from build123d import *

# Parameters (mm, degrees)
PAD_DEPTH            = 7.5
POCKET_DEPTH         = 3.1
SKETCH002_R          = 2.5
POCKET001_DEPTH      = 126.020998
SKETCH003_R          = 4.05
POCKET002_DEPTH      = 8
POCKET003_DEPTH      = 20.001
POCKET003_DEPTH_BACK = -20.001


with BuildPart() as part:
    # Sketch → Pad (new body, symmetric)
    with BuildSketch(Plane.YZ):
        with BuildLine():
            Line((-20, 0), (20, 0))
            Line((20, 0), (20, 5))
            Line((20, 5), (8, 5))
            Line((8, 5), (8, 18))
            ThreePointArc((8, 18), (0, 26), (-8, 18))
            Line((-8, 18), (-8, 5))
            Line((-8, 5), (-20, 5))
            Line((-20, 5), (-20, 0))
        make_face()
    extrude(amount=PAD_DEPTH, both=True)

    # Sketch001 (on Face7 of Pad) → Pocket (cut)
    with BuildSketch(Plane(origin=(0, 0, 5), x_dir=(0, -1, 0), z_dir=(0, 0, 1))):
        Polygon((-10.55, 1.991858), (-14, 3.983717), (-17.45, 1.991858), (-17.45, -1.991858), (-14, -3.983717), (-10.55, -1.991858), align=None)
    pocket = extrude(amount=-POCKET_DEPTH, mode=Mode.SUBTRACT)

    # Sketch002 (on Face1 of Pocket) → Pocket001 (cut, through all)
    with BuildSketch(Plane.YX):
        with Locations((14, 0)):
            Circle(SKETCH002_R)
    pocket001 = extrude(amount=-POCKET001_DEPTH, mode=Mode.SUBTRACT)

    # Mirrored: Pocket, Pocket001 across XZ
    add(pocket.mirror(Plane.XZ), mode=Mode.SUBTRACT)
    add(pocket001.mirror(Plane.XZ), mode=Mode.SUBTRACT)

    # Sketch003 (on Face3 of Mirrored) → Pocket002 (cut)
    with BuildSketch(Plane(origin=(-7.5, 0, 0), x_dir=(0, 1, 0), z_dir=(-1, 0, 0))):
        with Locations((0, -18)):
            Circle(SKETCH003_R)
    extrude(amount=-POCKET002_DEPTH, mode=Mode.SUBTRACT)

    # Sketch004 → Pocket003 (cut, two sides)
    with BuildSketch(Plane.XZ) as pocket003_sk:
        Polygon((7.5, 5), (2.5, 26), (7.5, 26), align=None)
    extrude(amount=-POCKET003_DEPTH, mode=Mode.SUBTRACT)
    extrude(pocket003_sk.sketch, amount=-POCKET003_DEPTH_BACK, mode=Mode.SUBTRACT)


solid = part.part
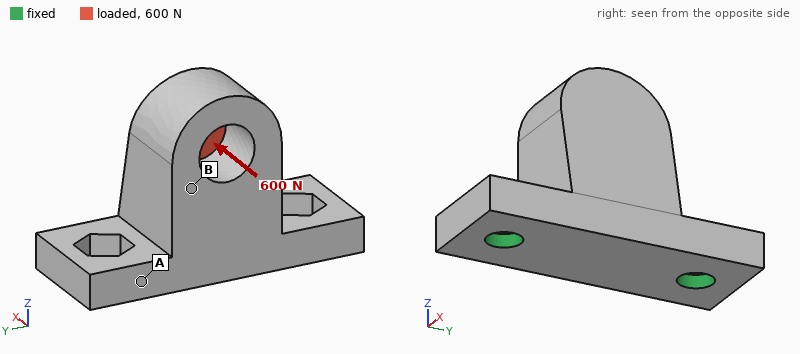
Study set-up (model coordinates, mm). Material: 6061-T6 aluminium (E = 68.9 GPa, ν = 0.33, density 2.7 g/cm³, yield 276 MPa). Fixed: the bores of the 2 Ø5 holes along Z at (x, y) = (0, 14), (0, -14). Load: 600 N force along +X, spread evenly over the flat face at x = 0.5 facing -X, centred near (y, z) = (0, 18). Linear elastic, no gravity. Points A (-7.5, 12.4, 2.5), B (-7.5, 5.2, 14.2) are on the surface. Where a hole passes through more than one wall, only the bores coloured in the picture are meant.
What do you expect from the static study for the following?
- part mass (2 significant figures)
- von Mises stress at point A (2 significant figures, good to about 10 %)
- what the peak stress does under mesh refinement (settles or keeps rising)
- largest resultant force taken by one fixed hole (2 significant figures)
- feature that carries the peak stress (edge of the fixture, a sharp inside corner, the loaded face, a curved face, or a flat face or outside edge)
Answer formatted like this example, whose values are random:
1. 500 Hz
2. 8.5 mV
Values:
1. 17 g
2. 49 MPa
3. keeps rising
4. 300 N
5. edge of the fixture
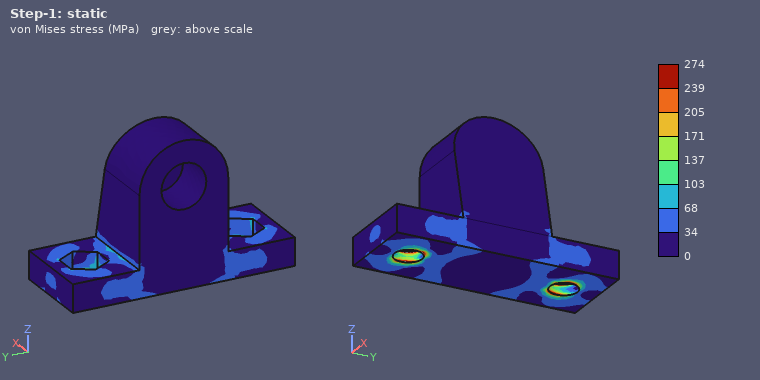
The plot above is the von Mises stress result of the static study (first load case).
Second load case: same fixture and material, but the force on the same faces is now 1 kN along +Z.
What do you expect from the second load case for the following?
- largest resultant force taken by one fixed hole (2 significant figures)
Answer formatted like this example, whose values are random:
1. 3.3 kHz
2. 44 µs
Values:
1. 630 N
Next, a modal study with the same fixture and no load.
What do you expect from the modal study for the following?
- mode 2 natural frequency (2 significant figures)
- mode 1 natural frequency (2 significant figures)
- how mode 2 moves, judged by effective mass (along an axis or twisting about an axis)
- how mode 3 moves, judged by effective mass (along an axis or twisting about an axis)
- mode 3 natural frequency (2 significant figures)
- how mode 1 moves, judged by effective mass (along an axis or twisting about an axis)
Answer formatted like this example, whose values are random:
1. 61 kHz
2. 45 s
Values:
1. 15 kHz
2. 5000 Hz
3. along Y
4. along Z
5. 17 kHz
6. along X
